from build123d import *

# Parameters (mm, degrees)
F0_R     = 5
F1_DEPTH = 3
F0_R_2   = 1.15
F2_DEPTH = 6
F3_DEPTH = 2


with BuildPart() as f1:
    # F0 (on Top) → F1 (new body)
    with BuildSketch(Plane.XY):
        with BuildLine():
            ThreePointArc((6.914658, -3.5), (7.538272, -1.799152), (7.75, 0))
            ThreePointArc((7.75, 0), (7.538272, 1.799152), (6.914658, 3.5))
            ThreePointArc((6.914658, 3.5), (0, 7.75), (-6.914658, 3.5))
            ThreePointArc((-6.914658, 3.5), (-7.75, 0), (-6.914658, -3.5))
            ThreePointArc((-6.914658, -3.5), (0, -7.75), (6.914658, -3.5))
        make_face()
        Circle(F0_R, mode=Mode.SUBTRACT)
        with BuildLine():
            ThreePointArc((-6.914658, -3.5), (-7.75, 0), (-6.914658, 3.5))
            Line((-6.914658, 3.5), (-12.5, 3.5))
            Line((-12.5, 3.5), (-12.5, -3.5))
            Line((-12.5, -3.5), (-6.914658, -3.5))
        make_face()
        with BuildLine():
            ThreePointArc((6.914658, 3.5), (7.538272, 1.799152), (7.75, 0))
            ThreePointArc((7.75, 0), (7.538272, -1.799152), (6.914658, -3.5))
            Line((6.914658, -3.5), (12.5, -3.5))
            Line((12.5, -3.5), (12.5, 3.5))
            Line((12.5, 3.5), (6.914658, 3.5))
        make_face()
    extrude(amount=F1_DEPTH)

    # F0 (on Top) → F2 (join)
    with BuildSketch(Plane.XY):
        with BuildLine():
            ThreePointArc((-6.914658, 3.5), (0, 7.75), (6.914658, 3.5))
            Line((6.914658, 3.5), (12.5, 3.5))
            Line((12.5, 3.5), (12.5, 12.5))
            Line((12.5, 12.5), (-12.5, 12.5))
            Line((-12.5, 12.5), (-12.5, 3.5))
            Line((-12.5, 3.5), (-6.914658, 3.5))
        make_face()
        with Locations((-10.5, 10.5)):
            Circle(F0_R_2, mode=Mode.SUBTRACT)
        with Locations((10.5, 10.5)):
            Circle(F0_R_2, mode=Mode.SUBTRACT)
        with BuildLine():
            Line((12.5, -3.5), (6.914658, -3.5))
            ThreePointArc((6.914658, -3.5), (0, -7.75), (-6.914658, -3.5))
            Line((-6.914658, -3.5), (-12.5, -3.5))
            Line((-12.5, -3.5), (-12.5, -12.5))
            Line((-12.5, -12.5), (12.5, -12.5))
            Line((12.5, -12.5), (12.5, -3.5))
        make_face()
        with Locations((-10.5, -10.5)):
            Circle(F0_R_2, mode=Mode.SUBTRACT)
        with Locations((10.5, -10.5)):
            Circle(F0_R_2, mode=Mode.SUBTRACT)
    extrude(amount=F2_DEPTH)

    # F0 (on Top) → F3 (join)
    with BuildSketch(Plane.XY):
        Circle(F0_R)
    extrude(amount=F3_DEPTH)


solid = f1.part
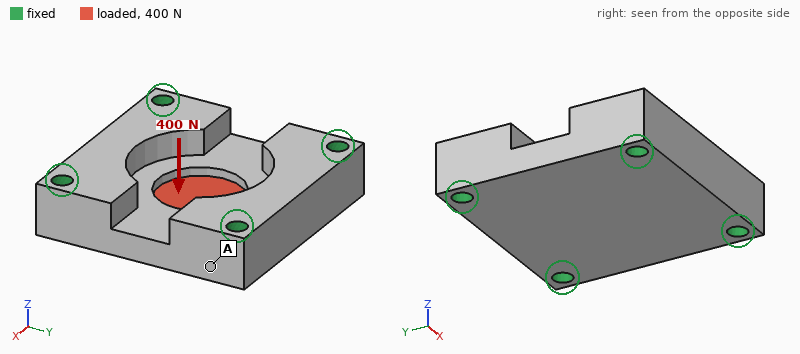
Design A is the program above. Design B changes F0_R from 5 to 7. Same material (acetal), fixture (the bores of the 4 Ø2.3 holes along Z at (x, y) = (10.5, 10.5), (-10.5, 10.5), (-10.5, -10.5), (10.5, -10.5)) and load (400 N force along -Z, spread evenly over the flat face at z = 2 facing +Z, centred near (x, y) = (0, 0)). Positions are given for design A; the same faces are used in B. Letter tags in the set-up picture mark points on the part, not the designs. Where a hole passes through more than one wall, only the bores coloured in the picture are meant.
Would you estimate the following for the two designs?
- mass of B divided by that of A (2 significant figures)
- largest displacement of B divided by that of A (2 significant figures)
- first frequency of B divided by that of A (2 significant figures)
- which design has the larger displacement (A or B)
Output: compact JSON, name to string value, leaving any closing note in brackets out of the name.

{"mass of B divided by that of A": "0.97", "largest displacement of B divided by that of A": "0.88", "first frequency of B divided by that of A": "1.0", "which design has the larger displacement": "A"}
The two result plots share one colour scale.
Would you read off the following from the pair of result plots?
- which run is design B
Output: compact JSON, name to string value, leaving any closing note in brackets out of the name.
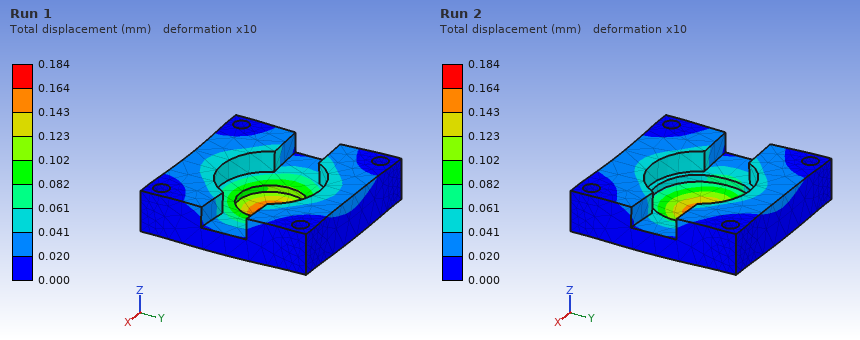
{"which run is design B": "Run 2"}
